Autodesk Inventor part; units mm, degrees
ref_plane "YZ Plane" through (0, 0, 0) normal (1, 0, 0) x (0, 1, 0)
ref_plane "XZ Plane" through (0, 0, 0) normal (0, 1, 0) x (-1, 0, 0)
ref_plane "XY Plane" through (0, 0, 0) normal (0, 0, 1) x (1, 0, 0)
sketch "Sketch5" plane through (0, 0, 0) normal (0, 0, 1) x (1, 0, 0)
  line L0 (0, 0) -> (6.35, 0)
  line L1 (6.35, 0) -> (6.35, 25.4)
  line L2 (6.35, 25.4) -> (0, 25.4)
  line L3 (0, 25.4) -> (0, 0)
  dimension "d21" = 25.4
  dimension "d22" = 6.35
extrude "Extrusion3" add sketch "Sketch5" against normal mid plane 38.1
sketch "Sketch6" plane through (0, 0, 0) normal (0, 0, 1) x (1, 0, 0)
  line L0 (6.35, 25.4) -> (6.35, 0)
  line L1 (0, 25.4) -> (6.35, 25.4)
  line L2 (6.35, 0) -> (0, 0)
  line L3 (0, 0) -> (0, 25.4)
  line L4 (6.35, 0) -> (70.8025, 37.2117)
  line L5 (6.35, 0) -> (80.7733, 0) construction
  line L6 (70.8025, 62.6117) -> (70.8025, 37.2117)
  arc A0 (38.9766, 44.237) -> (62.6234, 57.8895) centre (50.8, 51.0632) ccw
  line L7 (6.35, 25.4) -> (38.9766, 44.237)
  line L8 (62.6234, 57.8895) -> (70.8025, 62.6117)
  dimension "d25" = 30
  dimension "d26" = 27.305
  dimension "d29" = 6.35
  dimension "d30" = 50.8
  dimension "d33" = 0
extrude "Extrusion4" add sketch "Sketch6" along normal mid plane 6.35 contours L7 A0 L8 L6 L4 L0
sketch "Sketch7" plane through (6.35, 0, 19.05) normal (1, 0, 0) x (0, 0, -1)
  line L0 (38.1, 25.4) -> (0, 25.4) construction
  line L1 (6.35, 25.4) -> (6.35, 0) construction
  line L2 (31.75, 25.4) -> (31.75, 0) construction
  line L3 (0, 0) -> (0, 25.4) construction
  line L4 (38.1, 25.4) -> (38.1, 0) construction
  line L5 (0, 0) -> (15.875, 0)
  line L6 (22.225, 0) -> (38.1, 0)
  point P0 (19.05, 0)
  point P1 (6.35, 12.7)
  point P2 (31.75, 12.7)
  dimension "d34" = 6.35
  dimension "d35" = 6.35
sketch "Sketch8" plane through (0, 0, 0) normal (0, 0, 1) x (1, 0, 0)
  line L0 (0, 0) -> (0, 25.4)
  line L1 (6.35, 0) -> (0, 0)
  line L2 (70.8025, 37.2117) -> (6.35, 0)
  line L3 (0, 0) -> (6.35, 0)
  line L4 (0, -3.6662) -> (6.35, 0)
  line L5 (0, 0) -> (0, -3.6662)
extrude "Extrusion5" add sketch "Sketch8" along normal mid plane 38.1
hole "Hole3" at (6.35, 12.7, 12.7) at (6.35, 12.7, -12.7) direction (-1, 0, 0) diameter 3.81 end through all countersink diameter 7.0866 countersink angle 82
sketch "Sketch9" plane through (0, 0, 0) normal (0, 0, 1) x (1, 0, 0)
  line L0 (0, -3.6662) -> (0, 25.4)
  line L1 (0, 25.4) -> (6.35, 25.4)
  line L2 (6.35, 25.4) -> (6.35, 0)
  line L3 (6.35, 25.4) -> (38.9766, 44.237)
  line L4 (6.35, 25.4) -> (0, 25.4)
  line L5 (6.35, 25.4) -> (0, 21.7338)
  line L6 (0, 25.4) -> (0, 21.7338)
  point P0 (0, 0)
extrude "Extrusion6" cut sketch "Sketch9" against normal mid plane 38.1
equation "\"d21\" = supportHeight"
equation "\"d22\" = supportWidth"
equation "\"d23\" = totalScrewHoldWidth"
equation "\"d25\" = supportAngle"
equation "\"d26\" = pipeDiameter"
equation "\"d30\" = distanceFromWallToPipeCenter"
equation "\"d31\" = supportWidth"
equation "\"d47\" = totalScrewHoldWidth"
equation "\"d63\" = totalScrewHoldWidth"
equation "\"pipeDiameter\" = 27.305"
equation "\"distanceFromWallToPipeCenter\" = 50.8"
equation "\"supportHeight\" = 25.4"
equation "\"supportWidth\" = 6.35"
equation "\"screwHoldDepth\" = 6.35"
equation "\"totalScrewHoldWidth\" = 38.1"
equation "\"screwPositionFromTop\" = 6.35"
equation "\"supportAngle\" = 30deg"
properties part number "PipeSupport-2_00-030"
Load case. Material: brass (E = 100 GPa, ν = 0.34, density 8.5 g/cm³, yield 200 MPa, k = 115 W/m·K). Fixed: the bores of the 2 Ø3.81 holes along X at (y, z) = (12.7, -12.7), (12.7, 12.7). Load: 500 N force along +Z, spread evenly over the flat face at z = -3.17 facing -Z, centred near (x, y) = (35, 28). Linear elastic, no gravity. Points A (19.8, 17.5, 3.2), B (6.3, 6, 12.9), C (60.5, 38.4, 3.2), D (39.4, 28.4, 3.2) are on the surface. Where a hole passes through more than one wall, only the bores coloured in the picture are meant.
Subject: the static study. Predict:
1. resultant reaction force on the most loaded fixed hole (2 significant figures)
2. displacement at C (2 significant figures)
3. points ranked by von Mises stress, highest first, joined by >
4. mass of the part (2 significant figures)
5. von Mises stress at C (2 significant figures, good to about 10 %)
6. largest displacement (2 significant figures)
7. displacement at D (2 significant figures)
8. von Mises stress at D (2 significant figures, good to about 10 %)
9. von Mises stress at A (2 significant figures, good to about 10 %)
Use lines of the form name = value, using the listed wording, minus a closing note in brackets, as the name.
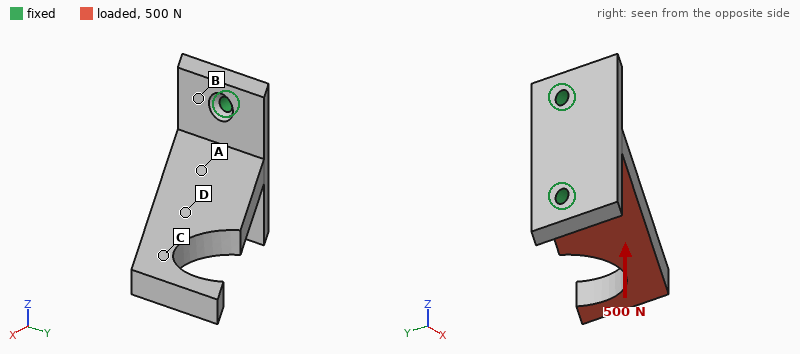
resultant reaction force on the most loaded fixed hole = 840 N
displacement at C = 0.38 mm
points ranked by von Mises stress, highest first, joined by > = A > D > C > B
mass of the part = 120 g
von Mises stress at C = 15 MPa
largest displacement = 0.58 mm
displacement at D = 0.18 mm
von Mises stress at D = 29 MPa
von Mises stress at A = 65 MPa
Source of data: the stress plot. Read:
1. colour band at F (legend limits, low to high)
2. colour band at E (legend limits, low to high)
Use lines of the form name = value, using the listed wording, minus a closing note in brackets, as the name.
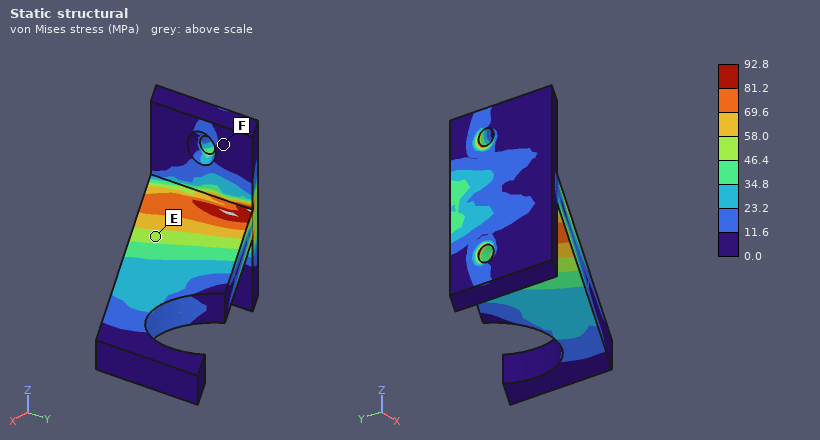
colour band at F = 0.0 to 11.6 MPa
colour band at E = 46.4 to 58.0 MPa
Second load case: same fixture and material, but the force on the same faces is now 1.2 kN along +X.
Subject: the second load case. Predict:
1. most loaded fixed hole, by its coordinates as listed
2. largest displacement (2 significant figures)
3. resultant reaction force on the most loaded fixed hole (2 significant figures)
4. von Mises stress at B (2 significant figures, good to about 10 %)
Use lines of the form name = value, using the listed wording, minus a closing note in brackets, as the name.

most loaded fixed hole, by its coordinates as listed = (12.7, -12.7)
largest displacement = 0.30 mm
resultant reaction force on the most loaded fixed hole = 870 N
von Mises stress at B = 26 MPa
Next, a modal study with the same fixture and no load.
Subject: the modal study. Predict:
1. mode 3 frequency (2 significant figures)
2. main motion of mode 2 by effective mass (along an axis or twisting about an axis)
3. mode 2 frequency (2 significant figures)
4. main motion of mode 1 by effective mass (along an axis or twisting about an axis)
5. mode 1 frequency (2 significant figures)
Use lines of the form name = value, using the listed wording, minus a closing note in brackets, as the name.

mode 3 frequency = 2900 Hz
main motion of mode 2 by effective mass = along Y
mode 2 frequency = 1200 Hz
main motion of mode 1 by effective mass = along Z
mode 1 frequency = 730 Hz
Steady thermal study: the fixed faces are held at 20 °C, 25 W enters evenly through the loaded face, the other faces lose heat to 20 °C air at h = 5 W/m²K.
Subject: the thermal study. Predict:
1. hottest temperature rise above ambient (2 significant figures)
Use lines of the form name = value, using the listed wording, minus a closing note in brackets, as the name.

hottest temperature rise above ambient = 72 K
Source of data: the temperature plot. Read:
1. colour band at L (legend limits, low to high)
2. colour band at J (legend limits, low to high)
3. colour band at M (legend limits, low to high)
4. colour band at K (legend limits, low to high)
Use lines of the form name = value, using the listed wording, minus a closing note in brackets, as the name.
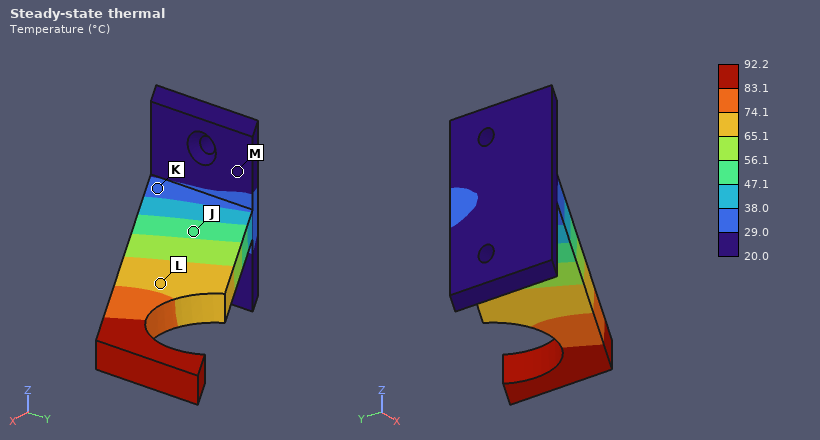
colour band at L = 65.1 to 74.1 °C
colour band at J = 47.1 to 56.1 °C
colour band at M = 20.0 to 29.0 °C
colour band at K = 29.0 to 38.0 °C
